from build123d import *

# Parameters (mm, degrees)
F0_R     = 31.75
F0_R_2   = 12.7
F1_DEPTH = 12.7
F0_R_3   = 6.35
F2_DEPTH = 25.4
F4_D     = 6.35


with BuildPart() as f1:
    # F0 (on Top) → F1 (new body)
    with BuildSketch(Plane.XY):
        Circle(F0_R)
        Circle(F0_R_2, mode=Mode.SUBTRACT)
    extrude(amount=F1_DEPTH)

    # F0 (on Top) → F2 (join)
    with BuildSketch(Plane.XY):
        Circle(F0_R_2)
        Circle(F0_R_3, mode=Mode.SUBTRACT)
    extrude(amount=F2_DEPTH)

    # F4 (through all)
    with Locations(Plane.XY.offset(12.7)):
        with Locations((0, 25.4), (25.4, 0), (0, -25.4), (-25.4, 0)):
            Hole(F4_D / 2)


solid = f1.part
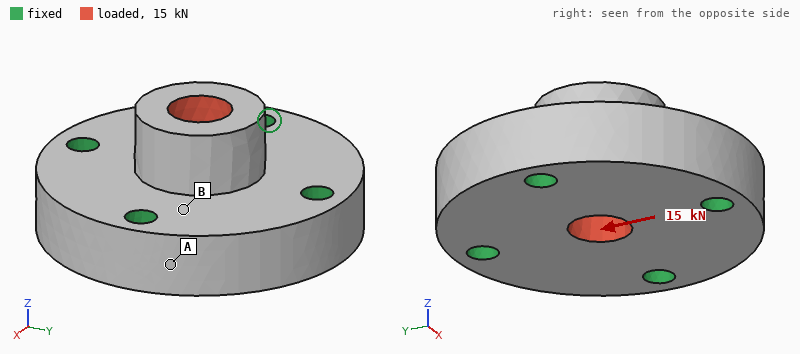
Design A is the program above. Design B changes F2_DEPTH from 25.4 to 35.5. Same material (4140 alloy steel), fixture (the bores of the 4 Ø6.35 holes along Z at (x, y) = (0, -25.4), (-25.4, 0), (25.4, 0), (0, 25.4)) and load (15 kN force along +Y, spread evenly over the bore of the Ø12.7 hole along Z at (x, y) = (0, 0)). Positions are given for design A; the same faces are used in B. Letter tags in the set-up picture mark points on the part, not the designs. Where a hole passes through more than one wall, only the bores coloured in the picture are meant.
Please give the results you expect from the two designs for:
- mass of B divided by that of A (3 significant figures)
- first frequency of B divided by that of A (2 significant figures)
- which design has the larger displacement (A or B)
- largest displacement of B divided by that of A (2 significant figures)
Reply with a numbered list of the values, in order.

1. 1.09
2. 0.62
3. B
4. 2.5
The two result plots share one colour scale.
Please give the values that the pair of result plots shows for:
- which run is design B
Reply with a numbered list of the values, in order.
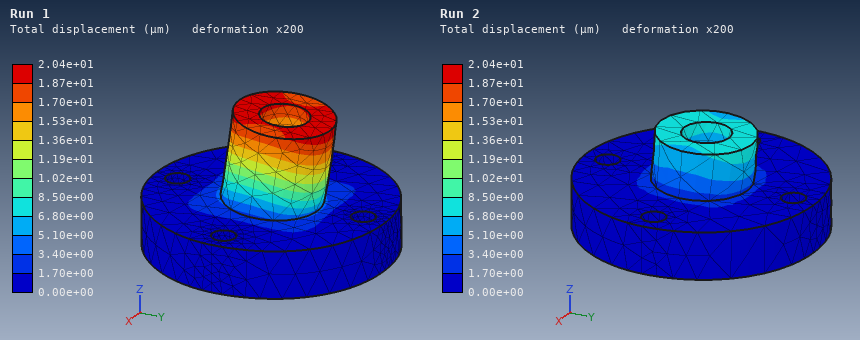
1. Run 1
